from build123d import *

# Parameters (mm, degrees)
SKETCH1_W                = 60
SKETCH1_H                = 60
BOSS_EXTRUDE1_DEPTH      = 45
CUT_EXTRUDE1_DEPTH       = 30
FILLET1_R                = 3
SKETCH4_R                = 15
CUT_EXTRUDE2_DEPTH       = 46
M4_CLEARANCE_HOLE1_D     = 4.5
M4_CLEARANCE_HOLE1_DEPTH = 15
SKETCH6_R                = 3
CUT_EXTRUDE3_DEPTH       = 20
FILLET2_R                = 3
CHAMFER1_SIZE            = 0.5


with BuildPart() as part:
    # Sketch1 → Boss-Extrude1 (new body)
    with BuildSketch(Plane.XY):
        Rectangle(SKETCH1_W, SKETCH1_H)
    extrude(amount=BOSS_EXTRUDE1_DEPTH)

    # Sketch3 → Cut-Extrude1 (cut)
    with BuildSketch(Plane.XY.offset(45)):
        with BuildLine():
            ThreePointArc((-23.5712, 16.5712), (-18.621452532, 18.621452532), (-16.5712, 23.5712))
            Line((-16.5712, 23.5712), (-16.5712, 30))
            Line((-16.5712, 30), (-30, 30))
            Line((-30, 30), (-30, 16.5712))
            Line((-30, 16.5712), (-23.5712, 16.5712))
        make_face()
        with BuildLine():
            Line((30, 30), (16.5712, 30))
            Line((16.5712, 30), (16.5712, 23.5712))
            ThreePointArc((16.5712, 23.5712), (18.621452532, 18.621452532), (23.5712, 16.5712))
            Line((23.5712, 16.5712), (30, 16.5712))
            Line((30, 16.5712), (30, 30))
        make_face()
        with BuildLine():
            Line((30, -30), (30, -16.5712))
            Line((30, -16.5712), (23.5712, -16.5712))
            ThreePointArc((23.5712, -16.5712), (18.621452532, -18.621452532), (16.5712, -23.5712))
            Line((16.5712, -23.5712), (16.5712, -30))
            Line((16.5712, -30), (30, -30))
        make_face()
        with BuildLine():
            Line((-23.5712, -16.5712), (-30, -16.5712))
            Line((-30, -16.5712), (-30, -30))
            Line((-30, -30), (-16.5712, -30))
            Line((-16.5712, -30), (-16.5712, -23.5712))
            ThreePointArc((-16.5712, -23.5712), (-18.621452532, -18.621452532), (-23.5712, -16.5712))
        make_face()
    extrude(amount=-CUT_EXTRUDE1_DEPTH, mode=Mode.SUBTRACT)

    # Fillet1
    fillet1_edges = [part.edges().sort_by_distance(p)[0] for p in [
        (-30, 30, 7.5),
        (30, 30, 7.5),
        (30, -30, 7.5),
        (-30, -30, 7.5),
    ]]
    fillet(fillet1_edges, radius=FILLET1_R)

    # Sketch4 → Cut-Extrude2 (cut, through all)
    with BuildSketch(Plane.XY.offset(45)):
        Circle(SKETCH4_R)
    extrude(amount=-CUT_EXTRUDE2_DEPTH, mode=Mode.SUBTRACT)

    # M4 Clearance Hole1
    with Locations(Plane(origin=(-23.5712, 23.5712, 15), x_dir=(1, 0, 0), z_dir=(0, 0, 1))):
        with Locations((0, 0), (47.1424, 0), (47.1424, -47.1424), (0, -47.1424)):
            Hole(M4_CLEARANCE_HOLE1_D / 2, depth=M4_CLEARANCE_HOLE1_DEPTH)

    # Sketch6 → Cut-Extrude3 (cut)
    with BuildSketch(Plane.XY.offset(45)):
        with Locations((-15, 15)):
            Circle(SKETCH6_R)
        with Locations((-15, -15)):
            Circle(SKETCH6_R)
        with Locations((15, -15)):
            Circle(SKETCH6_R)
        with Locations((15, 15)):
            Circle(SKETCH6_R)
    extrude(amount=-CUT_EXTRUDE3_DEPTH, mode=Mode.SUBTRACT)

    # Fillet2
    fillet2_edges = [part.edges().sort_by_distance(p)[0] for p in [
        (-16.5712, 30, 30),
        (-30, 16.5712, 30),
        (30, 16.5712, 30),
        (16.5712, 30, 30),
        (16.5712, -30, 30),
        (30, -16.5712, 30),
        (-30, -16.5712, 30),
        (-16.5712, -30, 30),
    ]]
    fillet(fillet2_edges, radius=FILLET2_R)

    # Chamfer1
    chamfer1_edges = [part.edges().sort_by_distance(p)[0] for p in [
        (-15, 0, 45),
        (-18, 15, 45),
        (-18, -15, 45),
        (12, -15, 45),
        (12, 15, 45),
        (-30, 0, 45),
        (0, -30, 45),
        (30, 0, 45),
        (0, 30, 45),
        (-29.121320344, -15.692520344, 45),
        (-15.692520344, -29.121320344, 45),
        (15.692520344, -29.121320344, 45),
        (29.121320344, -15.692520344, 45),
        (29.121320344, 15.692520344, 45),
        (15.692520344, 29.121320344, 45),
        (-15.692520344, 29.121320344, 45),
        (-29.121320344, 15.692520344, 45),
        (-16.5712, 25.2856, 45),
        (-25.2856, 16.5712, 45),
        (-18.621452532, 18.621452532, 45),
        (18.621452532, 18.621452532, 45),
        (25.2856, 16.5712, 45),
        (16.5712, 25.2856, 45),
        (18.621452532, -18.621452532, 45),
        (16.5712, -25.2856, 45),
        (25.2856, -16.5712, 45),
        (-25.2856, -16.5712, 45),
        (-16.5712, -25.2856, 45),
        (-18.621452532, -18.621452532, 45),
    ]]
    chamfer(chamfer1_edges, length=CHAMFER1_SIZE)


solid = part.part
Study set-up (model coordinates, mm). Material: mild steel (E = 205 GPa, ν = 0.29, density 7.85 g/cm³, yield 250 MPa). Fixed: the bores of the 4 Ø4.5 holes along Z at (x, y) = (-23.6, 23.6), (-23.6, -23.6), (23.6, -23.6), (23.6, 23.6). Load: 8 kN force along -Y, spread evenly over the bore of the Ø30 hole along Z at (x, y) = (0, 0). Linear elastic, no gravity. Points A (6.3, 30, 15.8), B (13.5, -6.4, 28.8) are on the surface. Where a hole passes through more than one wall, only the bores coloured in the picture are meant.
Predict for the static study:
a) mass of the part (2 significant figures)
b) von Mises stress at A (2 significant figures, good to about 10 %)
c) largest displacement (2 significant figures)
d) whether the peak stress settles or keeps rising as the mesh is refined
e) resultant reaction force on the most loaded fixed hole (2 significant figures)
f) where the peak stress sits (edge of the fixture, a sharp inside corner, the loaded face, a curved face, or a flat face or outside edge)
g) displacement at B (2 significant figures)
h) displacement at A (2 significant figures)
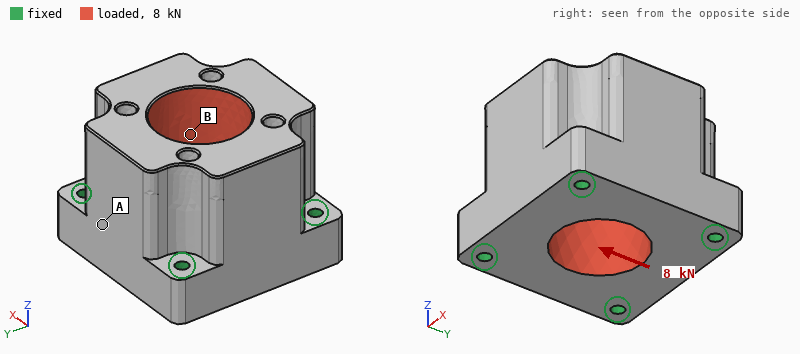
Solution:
830 g
2.9 MPa
3.0 µm
keeps rising
2.4 kN
edge of the fixture
1.9 µm
1.6 µm
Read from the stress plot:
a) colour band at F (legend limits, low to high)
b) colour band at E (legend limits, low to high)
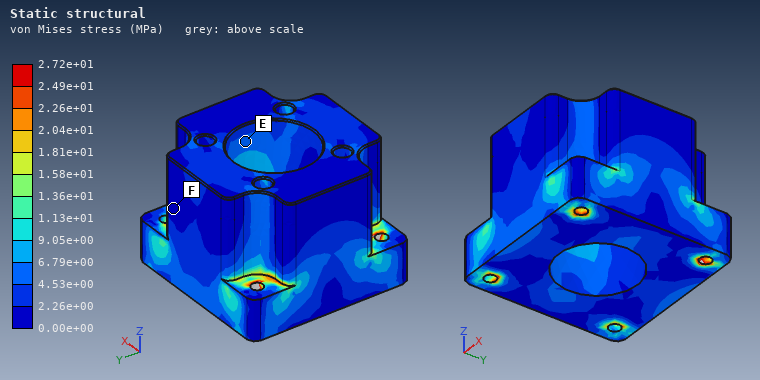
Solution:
0.00e+00 to 2.26e+00 MPa
4.53e+00 to 6.79e+00 MPa
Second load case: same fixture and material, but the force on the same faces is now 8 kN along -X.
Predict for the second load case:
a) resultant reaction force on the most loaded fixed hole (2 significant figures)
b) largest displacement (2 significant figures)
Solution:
2.4 kN
3.0 µm
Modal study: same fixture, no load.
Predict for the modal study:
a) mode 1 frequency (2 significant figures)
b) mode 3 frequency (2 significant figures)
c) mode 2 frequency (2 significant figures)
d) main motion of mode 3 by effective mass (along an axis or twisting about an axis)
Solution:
11 kHz
15 kHz
11 kHz
along Z
